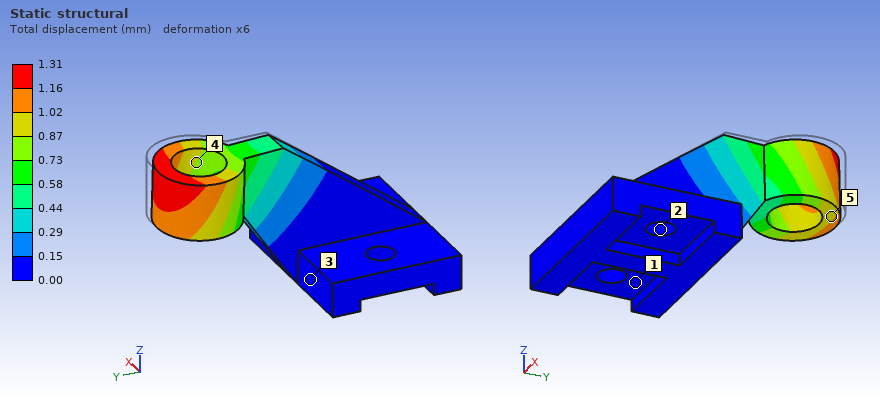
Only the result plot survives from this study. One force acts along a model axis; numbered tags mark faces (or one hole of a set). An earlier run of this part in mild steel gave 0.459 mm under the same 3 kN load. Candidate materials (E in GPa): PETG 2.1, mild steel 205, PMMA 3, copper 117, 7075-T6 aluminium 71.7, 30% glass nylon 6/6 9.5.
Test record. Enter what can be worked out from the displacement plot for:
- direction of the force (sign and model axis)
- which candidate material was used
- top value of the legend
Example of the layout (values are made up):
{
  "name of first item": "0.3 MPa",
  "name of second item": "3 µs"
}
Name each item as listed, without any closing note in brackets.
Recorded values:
{
  "direction of the force": "-X",
  "which candidate material was used": "7075-T6 aluminium",
  "top value of the legend": "1.31 mm"
}
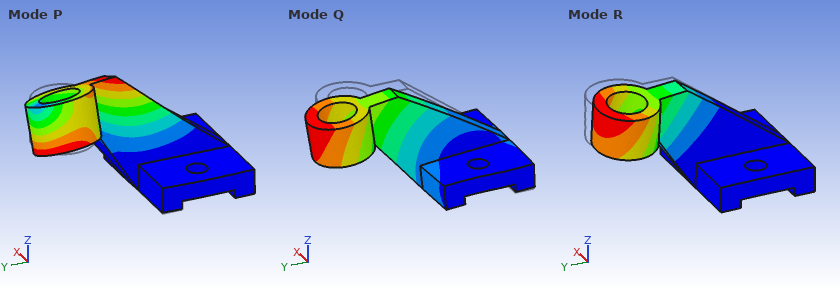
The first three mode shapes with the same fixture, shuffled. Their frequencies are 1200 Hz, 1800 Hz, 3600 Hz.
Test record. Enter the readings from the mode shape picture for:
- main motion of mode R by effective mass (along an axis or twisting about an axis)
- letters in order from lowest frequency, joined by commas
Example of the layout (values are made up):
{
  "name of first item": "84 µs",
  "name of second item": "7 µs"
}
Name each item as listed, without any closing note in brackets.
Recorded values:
{
  "main motion of mode R by effective mass": "along X",
  "letters in order from lowest frequency, joined by commas": "R, Q, P"
}
